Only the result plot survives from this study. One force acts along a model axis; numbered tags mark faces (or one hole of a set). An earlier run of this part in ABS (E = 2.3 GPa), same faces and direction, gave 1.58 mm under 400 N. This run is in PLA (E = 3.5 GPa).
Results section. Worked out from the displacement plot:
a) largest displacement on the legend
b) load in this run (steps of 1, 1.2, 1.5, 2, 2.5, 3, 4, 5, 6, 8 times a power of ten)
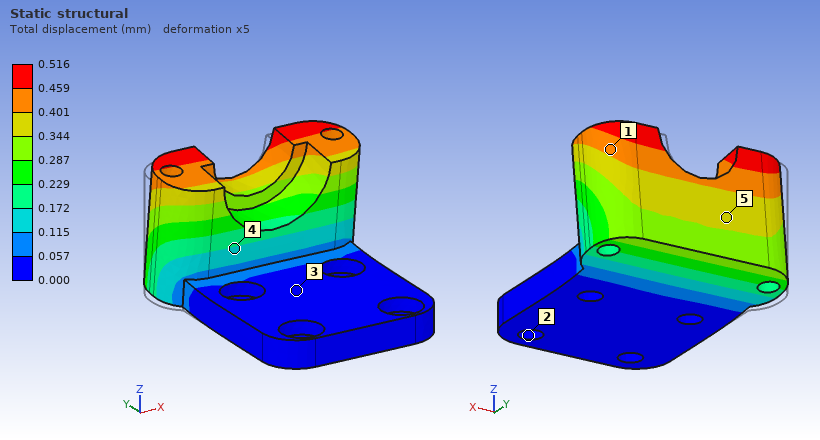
0.516 mm
200 N
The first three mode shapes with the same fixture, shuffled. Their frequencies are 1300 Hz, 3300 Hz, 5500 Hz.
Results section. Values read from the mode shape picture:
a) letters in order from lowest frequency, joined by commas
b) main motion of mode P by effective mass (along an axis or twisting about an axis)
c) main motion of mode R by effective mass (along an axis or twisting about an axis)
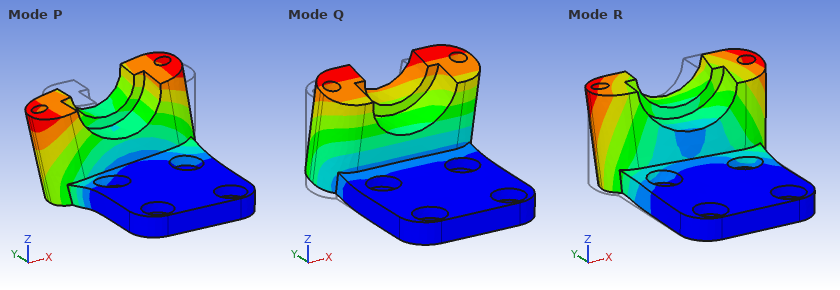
Q, P, R
along X
along X
